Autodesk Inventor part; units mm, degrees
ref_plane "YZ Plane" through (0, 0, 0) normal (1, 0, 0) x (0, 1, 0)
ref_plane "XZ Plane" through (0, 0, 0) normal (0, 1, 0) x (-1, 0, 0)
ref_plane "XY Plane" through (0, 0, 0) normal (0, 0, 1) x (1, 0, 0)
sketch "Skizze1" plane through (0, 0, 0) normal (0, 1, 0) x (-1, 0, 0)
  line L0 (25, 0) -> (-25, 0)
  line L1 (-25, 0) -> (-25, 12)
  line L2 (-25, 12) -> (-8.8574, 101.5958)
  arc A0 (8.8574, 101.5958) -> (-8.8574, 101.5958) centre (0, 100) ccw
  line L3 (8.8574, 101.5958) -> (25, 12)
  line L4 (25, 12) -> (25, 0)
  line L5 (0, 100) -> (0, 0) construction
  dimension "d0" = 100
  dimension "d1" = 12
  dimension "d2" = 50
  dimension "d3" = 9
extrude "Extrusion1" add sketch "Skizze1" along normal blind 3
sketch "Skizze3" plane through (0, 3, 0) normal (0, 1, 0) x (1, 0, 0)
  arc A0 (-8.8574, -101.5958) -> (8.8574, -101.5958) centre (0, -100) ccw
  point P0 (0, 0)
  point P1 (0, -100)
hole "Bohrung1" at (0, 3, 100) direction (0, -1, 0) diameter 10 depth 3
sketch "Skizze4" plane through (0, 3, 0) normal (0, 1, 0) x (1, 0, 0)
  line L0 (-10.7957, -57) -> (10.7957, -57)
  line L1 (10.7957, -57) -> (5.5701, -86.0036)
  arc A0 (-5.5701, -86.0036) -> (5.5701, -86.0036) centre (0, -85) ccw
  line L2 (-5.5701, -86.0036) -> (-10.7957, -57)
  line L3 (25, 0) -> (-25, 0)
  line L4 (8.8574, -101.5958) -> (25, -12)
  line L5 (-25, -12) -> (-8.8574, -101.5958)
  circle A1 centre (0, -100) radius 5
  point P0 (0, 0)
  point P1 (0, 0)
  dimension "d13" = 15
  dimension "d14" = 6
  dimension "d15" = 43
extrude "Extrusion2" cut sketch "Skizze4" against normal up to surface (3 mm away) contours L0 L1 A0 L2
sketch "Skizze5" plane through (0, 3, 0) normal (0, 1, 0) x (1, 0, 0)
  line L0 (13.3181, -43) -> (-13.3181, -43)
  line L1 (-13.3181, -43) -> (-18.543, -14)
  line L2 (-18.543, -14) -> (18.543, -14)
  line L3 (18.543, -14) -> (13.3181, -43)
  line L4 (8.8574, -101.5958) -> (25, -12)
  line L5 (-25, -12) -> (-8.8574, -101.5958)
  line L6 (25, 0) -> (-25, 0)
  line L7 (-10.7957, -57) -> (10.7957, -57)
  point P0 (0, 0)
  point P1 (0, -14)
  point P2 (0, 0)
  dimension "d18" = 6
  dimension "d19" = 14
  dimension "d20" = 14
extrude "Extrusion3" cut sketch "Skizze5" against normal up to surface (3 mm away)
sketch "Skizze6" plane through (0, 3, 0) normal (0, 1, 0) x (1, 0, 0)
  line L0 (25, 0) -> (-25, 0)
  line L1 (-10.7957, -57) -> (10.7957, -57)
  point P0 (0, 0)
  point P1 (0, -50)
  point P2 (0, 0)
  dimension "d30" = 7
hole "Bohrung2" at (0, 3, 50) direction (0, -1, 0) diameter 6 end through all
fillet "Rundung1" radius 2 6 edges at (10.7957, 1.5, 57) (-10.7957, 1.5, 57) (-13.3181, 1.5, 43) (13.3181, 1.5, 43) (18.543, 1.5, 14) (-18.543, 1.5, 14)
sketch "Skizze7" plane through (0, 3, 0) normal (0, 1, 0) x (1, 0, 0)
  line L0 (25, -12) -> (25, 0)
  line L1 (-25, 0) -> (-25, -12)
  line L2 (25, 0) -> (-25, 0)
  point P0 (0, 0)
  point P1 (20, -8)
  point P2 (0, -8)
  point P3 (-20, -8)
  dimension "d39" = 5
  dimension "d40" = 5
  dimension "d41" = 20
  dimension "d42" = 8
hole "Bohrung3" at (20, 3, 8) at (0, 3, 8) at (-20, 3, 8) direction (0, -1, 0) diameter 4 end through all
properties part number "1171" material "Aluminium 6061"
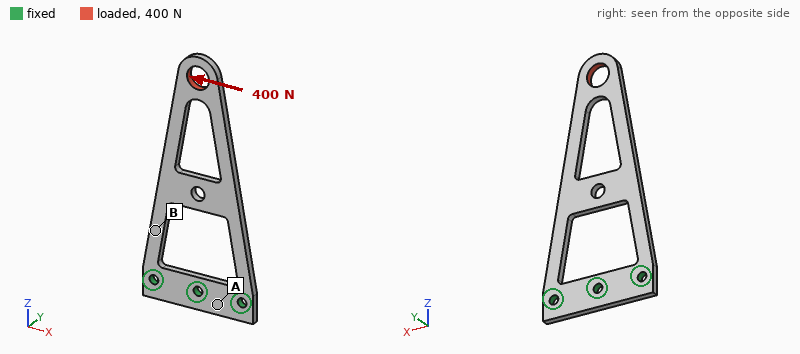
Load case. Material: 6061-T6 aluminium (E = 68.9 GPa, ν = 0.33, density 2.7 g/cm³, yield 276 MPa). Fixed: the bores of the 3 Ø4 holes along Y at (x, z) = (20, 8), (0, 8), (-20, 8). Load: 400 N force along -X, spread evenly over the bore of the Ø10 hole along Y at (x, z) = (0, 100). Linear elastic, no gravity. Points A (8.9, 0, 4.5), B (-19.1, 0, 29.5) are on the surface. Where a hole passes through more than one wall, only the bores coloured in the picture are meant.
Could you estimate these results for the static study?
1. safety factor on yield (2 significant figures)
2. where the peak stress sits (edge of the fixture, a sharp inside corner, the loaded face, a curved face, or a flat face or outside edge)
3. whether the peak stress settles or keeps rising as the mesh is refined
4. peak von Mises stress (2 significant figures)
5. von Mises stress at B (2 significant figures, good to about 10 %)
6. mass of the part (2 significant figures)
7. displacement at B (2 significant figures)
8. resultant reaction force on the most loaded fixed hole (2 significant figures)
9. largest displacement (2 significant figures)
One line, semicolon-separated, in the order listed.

1.9; a curved face; settles; 140 MPa; 44 MPa; 17 g; 0.050 mm; 850 N; 0.28 mm
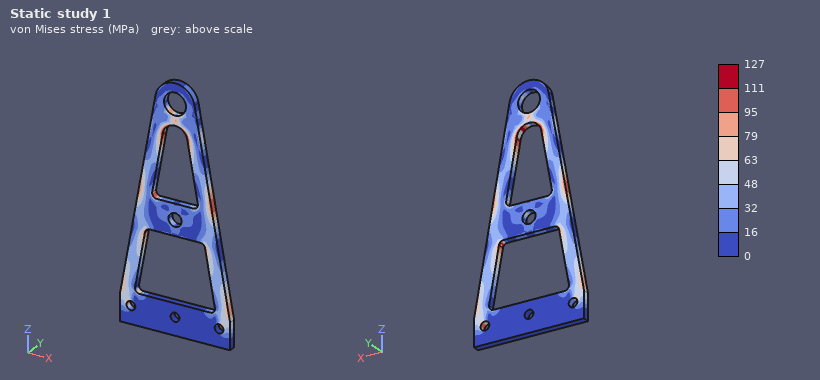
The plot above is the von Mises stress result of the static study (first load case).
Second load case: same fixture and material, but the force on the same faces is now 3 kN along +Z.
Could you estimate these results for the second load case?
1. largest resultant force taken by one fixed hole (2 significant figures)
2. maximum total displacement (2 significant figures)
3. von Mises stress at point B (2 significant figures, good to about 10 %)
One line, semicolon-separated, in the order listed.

1.6 kN; 0.12 mm; 83 MPa
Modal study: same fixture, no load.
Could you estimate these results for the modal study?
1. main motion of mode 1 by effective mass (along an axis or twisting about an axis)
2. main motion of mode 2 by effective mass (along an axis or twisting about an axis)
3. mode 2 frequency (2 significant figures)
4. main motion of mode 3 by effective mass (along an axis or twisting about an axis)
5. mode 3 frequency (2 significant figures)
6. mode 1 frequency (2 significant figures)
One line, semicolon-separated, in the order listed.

along Y; along Y; 1400 Hz; twisting about Z; 1600 Hz; 250 Hz
